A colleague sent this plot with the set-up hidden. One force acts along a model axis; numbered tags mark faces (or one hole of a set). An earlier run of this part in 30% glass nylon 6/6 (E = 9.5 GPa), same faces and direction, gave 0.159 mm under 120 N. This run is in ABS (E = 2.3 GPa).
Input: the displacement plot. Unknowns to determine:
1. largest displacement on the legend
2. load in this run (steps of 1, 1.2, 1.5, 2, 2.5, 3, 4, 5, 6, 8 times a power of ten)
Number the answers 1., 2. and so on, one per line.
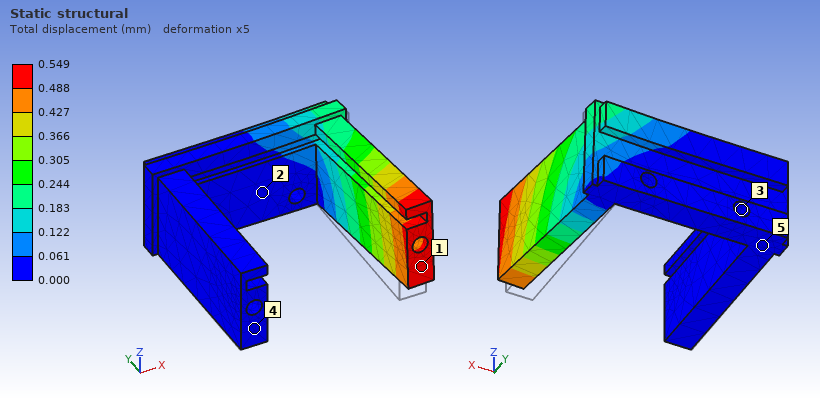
1. 0.549 mm
2. 100 N
